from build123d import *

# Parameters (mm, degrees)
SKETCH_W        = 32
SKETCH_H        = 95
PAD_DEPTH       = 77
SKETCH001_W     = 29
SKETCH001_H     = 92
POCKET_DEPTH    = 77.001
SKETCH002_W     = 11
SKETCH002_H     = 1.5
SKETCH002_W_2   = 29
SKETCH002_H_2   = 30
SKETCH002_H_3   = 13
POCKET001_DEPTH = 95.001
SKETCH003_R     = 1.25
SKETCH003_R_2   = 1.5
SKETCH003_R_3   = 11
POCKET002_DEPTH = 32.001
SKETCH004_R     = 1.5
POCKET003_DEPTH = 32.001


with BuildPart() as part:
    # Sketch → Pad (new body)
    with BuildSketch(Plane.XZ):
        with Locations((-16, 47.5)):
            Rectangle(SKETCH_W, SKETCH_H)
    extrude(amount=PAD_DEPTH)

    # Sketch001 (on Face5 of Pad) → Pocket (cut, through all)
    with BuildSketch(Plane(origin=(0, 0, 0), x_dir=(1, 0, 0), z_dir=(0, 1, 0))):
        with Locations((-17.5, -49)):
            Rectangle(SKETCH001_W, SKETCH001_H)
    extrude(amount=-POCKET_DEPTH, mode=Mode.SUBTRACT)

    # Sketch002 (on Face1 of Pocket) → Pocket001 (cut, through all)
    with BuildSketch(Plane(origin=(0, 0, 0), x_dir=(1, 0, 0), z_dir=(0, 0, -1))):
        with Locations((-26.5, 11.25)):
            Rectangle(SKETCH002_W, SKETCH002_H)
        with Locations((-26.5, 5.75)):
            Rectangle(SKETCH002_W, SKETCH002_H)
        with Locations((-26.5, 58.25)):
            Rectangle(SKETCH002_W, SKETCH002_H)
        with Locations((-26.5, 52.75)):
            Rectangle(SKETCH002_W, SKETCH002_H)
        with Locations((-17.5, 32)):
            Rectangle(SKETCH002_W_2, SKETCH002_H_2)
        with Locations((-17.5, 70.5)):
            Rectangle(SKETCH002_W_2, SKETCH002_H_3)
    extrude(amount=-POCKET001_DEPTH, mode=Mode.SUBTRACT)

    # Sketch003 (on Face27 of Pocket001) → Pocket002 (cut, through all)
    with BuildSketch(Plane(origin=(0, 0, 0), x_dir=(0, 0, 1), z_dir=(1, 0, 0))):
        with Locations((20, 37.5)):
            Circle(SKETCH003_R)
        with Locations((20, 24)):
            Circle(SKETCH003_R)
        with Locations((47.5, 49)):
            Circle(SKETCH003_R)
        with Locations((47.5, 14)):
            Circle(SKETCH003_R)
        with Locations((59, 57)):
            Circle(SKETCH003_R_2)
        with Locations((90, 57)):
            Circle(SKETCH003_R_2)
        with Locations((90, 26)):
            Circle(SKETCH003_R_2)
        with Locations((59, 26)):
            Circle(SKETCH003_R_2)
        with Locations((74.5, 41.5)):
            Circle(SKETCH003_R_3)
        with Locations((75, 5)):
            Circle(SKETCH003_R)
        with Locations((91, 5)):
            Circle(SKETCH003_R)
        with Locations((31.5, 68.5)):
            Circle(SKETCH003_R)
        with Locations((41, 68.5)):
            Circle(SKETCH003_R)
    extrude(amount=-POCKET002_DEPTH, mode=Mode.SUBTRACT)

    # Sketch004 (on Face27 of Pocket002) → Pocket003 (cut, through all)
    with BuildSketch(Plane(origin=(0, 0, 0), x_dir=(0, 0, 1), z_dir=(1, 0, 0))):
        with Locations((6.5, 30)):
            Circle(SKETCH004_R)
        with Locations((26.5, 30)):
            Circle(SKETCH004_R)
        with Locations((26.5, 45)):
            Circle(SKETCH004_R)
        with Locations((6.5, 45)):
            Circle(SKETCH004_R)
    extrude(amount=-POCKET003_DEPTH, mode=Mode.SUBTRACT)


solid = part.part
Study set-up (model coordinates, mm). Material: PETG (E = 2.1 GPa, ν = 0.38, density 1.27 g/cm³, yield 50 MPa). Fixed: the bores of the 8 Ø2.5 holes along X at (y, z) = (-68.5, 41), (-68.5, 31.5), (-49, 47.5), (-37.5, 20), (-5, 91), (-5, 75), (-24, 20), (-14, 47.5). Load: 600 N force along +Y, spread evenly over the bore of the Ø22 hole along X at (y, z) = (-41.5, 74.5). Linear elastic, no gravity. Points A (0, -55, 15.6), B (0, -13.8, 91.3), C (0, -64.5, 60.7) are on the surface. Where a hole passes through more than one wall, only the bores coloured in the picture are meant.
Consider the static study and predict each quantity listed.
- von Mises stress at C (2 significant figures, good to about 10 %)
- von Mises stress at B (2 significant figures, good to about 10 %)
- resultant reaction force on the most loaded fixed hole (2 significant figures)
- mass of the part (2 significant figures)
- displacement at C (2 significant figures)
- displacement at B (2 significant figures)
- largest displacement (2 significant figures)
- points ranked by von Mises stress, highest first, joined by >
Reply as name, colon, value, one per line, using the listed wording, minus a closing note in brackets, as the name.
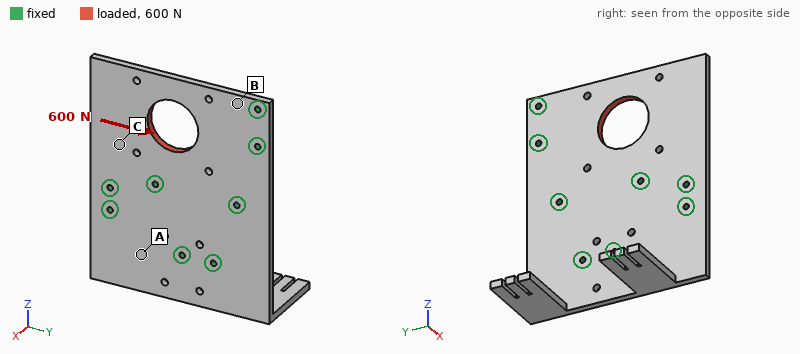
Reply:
von Mises stress at C: 2.9 MPa
von Mises stress at B: 5.1 MPa
resultant reaction force on the most loaded fixed hole: 160 N
mass of the part: 30 g
displacement at C: 0.051 mm
displacement at B: 0.025 mm
largest displacement: 0.12 mm
points ranked by von Mises stress, highest first, joined by >: B > C > A
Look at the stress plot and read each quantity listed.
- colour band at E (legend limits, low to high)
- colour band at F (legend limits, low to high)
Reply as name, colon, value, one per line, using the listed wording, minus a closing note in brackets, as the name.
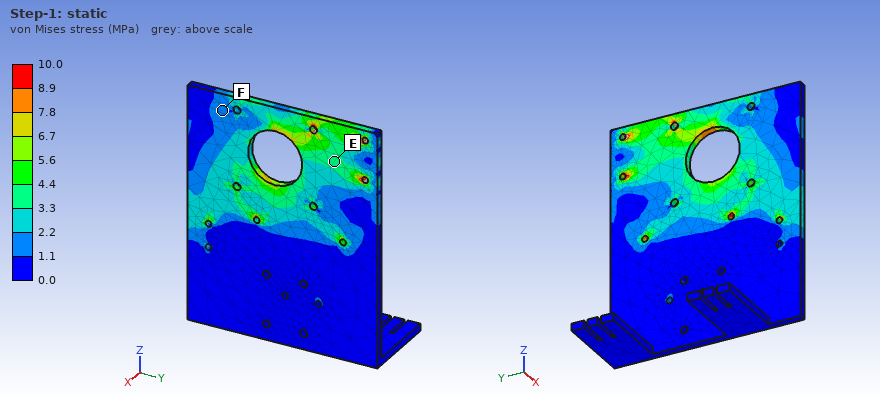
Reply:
colour band at E: 3.3 to 4.4 MPa
colour band at F: 1.1 to 2.2 MPa
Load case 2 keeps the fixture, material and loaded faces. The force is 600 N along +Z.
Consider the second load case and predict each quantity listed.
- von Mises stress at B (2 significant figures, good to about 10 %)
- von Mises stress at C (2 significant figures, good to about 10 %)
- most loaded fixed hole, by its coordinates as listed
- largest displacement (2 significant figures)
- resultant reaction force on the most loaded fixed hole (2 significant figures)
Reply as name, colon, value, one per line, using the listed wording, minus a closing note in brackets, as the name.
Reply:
von Mises stress at B: 2.1 MPa
von Mises stress at C: 3.0 MPa
most loaded fixed hole, by its coordinates as listed: (-49, 47.5)
largest displacement: 0.13 mm
resultant reaction force on the most loaded fixed hole: 170 N
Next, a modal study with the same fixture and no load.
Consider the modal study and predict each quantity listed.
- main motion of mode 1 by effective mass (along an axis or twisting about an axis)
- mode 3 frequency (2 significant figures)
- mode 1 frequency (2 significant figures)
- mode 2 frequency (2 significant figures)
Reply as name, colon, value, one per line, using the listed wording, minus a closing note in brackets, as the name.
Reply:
main motion of mode 1 by effective mass: along X
mode 3 frequency: 420 Hz
mode 1 frequency: 340 Hz
mode 2 frequency: 390 Hz
